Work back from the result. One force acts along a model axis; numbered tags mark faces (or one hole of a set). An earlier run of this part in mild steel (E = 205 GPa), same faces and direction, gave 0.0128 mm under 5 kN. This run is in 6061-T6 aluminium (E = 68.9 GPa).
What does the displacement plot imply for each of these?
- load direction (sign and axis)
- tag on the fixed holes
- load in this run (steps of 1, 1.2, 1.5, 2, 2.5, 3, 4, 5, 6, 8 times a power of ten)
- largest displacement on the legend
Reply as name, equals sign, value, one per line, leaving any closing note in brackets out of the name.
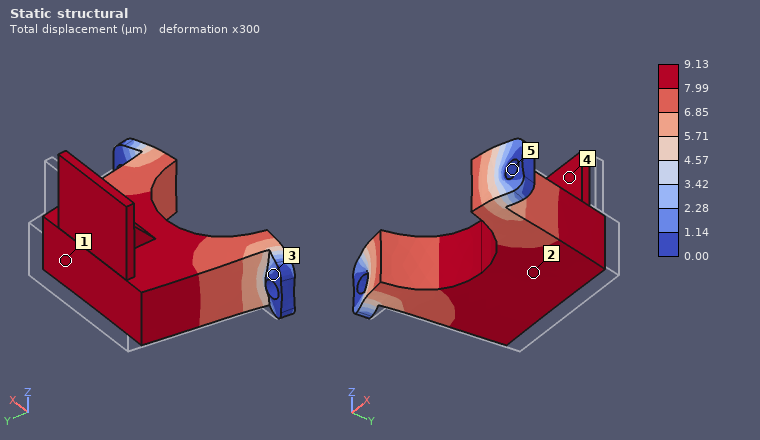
load direction = -Y
tag on the fixed holes = 5
load in this run = 1.2 kN
largest displacement on the legend = 9.13 µm
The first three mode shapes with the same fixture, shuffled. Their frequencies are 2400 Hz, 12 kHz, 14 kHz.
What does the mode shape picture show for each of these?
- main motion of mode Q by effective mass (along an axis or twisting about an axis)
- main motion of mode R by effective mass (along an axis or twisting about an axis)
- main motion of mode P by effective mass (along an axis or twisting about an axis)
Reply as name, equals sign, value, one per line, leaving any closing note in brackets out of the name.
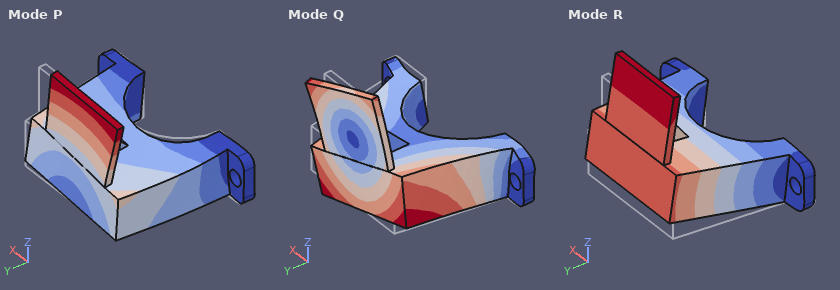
main motion of mode Q by effective mass = along X
main motion of mode R by effective mass = along Z
main motion of mode P by effective mass = along X
